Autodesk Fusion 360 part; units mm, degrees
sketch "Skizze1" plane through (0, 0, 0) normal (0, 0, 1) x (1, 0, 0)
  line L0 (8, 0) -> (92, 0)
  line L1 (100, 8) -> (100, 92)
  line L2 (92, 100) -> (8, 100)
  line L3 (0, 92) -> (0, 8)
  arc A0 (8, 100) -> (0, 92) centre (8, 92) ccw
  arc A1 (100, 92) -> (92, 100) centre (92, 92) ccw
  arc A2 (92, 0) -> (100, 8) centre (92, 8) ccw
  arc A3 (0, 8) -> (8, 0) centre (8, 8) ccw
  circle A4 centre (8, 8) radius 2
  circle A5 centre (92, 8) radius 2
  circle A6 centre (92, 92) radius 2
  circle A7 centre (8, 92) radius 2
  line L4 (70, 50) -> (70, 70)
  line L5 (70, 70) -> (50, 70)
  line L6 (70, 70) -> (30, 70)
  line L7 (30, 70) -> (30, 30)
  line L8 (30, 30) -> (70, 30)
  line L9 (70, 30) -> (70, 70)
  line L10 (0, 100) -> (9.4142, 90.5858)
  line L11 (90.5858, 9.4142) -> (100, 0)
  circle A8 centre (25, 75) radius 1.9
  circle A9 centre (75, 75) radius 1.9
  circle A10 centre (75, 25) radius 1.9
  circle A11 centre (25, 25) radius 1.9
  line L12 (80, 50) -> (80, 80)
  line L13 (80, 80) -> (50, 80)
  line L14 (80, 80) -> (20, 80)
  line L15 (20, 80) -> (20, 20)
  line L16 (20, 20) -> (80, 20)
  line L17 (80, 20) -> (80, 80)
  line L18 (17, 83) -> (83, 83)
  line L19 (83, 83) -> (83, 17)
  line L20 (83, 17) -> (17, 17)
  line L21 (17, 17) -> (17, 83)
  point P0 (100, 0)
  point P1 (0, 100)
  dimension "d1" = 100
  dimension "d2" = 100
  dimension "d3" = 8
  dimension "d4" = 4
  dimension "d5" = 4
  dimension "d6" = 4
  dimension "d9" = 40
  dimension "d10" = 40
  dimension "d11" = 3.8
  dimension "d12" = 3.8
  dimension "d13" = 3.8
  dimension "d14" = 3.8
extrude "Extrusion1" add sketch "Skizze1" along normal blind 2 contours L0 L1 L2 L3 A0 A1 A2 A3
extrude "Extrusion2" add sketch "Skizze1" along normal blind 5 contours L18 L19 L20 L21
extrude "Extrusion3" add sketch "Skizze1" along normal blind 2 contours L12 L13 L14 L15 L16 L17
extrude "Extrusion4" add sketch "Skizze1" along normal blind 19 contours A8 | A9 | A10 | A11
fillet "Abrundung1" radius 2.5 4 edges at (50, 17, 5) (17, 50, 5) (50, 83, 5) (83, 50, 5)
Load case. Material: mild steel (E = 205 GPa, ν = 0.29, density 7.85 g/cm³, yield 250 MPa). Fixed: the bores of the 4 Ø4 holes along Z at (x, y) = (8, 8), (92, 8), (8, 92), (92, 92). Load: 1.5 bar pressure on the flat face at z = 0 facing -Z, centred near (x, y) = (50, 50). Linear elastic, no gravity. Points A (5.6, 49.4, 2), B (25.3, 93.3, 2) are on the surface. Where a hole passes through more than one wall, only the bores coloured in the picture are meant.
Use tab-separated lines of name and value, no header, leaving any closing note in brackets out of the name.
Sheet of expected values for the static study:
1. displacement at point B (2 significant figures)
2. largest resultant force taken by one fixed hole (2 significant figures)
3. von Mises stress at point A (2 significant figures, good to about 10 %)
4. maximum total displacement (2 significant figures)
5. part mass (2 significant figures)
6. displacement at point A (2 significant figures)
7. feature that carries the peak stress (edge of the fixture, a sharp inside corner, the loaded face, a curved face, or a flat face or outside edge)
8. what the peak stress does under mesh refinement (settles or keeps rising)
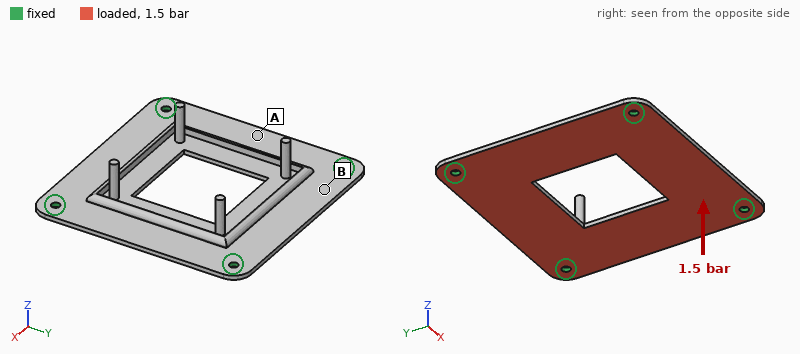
displacement at point B	0.049 mm
largest resultant force taken by one fixed hole	460 N
von Mises stress at point A	38 MPa
maximum total displacement	0.18 mm
part mass	150 g
displacement at point A	0.099 mm
feature that carries the peak stress	edge of the fixture
what the peak stress does under mesh refinement	keeps rising
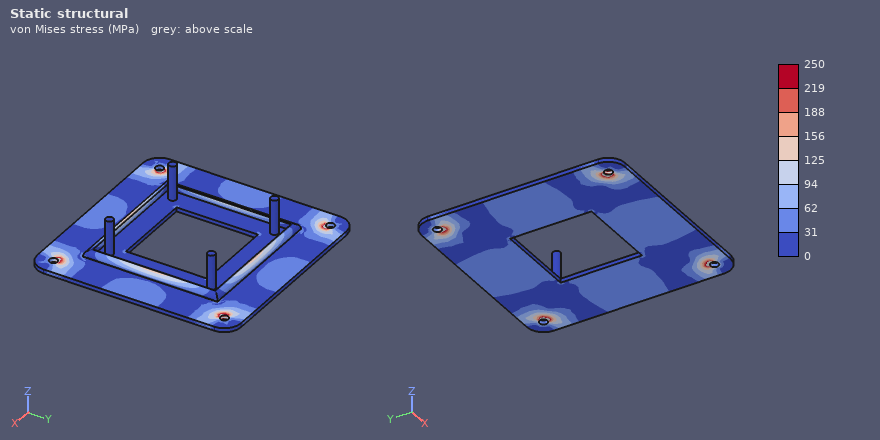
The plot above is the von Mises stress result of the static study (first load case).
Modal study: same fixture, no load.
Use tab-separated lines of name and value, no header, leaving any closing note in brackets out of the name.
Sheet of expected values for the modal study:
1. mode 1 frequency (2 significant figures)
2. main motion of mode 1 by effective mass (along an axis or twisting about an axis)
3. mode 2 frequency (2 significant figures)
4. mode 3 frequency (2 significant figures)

mode 1 frequency	1300 Hz
main motion of mode 1 by effective mass	along Z
mode 2 frequency	1900 Hz
mode 3 frequency	1900 Hz
